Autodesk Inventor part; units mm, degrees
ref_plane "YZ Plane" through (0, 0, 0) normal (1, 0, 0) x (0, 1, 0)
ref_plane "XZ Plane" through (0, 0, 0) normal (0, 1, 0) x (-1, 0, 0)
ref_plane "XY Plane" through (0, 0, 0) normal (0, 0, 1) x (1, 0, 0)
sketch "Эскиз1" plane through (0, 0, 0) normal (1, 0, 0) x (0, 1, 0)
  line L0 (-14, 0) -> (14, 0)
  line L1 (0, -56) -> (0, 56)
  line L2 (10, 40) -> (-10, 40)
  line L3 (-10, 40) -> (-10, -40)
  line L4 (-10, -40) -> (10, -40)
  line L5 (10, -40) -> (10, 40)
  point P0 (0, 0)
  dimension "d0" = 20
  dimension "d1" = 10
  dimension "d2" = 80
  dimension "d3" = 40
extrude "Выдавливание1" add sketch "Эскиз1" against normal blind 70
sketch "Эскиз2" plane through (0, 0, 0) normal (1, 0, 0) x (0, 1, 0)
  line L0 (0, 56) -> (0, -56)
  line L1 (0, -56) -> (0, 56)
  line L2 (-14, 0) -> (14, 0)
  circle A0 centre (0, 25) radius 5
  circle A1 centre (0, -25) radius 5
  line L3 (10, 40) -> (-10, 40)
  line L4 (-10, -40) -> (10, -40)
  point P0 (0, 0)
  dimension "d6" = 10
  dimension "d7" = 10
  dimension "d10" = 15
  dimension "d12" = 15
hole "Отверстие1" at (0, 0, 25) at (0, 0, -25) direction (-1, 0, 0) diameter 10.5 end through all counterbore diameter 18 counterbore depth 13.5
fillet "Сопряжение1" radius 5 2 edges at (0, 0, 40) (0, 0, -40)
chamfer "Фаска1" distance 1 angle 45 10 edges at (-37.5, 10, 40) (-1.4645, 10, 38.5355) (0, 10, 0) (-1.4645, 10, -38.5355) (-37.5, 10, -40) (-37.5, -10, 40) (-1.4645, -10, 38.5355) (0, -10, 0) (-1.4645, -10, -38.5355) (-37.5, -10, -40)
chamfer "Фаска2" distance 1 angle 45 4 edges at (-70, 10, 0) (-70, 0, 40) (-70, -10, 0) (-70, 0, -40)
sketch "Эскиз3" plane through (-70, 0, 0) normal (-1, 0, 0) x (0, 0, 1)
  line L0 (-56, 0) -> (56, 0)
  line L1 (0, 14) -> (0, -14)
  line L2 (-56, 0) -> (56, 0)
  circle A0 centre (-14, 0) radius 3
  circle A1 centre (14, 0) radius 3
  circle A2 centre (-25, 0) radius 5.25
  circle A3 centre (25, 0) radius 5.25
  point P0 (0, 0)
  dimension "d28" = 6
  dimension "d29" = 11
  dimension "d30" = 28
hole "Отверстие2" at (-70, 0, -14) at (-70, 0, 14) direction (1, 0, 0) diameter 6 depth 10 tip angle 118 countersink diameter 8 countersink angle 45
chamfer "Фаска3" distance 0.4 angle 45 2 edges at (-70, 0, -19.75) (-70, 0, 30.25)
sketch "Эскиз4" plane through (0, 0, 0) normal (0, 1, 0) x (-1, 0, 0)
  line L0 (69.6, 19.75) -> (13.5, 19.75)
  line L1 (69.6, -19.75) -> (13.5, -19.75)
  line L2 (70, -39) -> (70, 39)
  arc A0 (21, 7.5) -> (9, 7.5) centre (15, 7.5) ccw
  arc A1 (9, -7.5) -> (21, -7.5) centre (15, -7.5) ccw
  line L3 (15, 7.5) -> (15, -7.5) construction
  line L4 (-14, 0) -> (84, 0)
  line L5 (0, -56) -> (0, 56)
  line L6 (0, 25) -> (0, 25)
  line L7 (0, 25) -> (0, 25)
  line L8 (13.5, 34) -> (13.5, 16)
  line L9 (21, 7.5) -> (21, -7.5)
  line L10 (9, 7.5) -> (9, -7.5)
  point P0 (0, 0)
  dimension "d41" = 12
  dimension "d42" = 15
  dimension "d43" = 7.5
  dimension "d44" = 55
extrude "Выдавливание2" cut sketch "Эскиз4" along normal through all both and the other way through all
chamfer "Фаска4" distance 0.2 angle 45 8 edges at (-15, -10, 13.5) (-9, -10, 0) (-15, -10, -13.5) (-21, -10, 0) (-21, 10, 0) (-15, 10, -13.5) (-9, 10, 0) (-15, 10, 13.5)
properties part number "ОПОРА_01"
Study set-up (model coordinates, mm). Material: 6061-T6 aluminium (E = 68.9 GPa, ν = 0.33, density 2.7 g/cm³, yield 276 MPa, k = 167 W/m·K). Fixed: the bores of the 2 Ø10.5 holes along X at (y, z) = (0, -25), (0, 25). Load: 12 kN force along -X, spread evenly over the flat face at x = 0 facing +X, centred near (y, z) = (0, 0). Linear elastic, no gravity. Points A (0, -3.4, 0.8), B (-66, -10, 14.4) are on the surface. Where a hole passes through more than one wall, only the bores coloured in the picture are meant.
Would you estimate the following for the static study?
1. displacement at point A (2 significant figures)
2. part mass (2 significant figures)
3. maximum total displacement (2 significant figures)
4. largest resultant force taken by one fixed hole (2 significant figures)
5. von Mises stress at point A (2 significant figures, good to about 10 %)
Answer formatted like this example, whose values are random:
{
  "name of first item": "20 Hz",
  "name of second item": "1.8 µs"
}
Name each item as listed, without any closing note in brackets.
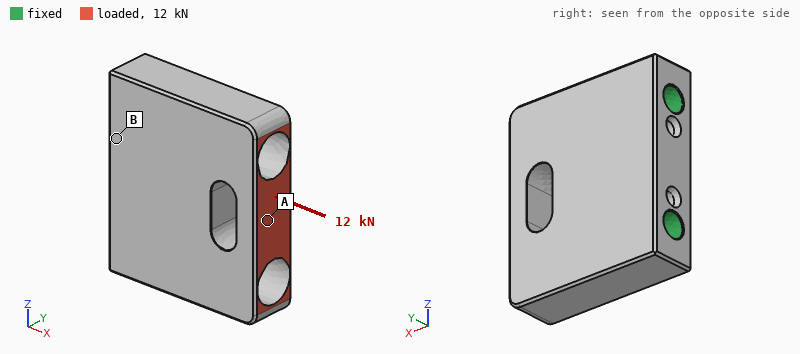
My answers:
{
  "displacement at point A": "24 µm",
  "part mass": "240 g",
  "maximum total displacement": "25 µm",
  "largest resultant force taken by one fixed hole": "6.6 kN",
  "von Mises stress at point A": "48 MPa"
}
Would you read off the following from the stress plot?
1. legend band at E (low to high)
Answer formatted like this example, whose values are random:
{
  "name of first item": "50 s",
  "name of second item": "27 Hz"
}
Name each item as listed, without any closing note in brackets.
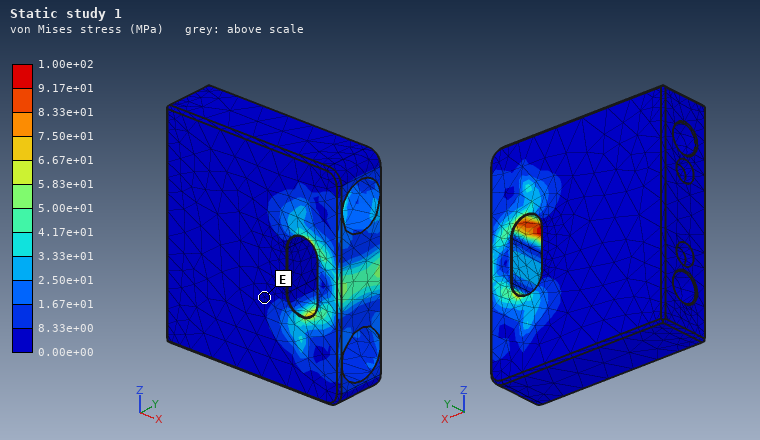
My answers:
{
  "legend band at E": "0.00e+00 to 8.33e+00 MPa"
}
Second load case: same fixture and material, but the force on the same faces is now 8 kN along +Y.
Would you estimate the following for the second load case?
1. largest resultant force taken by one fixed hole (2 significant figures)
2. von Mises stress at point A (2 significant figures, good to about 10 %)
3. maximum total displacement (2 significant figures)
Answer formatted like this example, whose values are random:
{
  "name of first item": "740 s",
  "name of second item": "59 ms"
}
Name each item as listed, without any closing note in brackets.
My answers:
{
  "largest resultant force taken by one fixed hole": "4.0 kN",
  "von Mises stress at point A": "21 MPa",
  "maximum total displacement": "68 µm"
}
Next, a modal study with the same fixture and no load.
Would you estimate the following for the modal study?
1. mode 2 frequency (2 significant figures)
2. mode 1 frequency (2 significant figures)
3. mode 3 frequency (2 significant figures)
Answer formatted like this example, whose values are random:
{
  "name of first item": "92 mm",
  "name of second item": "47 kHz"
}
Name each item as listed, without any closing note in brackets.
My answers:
{
  "mode 2 frequency": "23 kHz",
  "mode 1 frequency": "15 kHz",
  "mode 3 frequency": "24 kHz"
}
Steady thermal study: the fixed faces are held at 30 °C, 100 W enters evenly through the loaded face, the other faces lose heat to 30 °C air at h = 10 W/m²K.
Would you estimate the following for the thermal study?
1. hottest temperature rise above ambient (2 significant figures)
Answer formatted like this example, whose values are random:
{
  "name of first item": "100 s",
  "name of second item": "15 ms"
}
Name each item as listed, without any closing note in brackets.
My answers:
{
  "hottest temperature rise above ambient": "32 K"
}
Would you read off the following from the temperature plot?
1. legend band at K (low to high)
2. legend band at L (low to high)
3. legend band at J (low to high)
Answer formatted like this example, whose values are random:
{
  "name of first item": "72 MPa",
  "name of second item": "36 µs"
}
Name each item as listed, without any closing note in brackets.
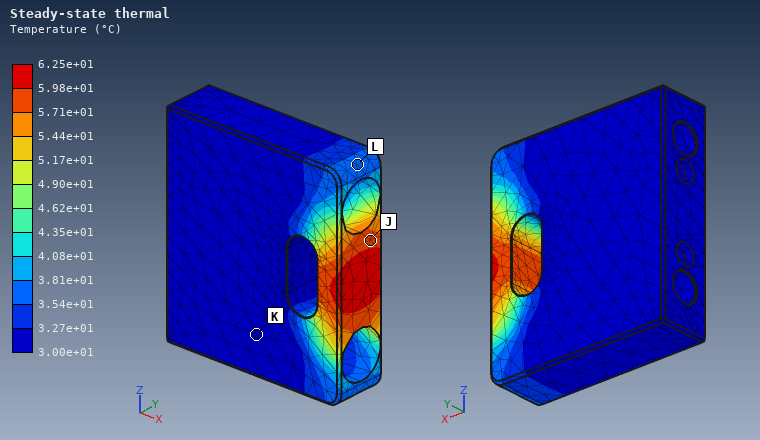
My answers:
{
  "legend band at K": "3.00e+01 to 3.27e+01 °C",
  "legend band at L": "3.54e+01 to 3.81e+01 °C",
  "legend band at J": "5.71e+01 to 5.98e+01 °C"
}
